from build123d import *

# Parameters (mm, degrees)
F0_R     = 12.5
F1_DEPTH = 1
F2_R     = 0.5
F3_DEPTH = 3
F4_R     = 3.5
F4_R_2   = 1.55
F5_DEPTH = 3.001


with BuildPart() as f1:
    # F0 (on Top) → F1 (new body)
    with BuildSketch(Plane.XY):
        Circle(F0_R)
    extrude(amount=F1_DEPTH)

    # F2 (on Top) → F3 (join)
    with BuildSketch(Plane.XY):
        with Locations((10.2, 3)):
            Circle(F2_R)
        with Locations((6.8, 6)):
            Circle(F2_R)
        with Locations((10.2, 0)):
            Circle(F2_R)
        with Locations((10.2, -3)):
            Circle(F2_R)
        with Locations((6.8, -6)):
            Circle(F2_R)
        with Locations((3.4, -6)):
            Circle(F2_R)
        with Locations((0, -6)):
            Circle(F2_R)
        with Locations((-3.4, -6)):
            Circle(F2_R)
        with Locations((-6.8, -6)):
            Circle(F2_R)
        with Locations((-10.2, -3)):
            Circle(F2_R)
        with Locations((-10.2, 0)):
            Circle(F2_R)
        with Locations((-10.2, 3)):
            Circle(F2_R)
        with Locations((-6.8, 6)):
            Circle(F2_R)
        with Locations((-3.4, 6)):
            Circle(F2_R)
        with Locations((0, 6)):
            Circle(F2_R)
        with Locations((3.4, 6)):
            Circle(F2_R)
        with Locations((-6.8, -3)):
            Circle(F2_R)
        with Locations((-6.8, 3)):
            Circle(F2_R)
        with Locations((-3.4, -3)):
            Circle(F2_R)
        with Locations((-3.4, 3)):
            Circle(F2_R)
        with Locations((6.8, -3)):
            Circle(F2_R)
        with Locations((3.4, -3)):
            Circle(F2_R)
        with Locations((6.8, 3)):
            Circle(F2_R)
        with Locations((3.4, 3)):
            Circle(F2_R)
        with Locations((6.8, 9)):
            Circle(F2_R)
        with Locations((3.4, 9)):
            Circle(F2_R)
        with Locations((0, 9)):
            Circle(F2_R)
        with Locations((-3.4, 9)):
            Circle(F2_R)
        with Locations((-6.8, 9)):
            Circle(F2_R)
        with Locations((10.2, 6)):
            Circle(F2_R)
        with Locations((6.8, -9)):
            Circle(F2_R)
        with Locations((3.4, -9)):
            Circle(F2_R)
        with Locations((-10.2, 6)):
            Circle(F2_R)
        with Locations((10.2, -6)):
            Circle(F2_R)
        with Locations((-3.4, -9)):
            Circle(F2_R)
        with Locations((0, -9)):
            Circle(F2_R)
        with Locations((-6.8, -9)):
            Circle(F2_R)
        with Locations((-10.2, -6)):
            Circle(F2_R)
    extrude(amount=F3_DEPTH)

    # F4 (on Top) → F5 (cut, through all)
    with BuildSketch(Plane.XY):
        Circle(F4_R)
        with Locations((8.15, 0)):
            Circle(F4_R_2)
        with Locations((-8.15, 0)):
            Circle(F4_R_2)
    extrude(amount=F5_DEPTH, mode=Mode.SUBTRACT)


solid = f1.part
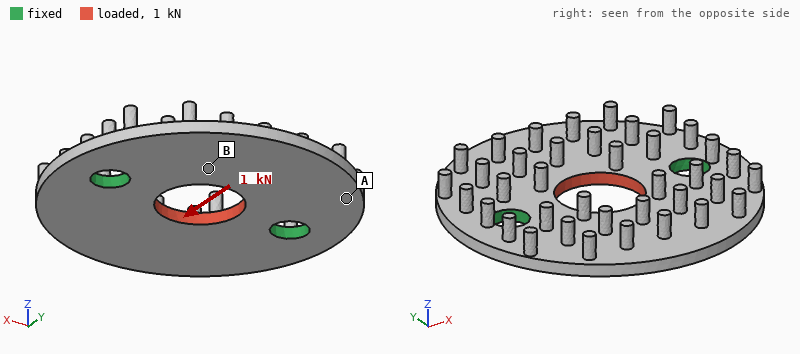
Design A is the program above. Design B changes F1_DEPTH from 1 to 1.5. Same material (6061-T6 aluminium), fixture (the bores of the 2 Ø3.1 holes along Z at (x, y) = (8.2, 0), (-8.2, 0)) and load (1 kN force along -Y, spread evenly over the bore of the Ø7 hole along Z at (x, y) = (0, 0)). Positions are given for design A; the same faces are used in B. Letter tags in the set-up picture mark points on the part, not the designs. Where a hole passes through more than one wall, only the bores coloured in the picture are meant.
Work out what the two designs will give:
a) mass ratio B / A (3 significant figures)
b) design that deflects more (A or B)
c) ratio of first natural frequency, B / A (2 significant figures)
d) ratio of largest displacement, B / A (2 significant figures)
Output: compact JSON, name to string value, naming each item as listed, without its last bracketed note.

{"mass ratio B / A": "1.41", "design that deflects more": "A", "ratio of first natural frequency, B / A": "1.5", "ratio of largest displacement, B / A": "0.67"}
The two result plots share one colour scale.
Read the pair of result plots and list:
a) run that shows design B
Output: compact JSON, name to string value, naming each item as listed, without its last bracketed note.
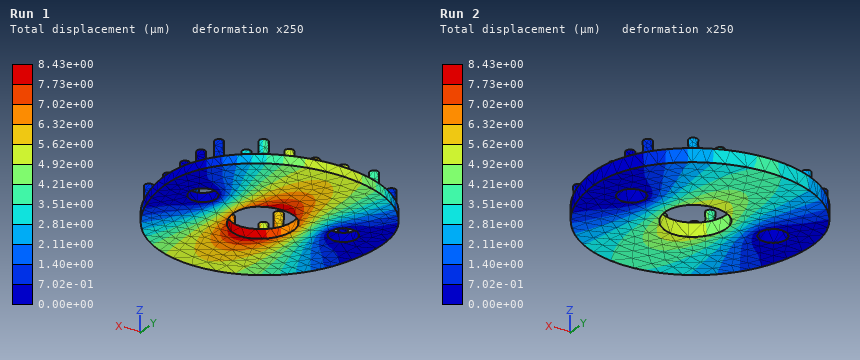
{"run that shows design B": "Run 2"}
